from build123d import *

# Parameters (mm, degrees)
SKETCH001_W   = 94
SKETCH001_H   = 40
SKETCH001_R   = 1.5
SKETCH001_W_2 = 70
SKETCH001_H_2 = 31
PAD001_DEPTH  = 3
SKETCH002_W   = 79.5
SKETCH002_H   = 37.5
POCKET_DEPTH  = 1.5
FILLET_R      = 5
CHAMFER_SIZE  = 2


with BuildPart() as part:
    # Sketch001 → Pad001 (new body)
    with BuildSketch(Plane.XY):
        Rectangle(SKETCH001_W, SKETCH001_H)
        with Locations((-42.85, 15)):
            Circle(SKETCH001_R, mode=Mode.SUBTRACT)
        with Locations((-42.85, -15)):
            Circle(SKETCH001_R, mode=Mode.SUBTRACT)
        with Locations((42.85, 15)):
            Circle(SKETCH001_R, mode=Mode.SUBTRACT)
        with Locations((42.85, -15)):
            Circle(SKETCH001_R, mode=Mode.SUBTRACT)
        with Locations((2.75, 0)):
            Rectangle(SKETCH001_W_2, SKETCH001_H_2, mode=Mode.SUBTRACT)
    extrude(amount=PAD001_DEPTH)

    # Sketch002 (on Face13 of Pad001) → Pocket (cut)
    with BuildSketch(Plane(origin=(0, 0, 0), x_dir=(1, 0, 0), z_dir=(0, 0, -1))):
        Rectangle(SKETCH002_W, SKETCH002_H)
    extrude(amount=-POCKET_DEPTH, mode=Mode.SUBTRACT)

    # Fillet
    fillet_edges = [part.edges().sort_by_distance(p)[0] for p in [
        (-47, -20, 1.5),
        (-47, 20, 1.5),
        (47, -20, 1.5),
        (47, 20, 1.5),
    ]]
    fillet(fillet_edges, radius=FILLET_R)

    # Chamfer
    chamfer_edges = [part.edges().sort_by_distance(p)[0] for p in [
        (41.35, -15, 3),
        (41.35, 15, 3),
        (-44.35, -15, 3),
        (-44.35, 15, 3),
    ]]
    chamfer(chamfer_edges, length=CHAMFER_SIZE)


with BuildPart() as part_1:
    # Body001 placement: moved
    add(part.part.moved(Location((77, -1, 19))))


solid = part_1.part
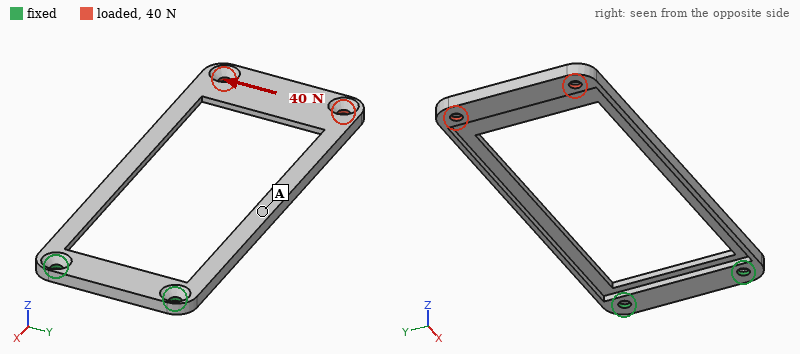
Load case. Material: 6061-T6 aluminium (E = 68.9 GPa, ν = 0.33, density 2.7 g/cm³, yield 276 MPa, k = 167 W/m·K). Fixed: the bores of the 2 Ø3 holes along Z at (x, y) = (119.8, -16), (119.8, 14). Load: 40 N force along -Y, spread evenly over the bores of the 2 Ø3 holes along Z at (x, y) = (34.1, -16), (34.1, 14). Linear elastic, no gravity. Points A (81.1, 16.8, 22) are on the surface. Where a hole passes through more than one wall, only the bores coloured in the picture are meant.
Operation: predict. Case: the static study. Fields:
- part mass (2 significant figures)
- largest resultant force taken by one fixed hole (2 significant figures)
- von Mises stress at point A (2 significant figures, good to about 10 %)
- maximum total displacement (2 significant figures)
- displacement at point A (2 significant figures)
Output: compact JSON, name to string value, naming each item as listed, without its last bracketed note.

{"part mass": "8.9 g", "largest resultant force taken by one fixed hole": "86 N", "von Mises stress at point A": "17 MPa", "maximum total displacement": "1.1 mm", "displacement at point A": "0.45 mm"}
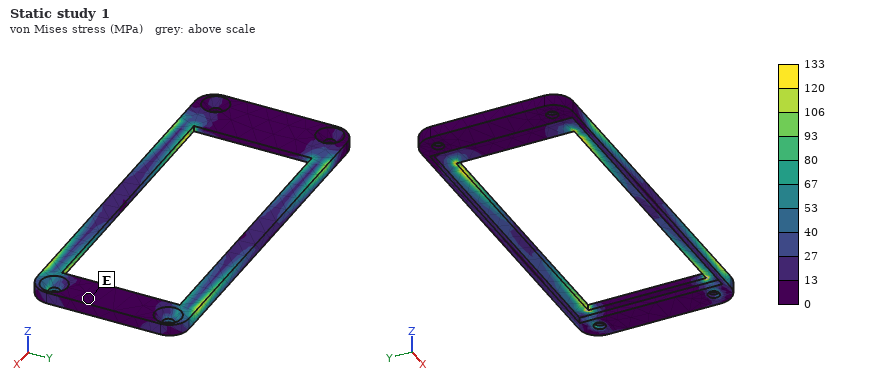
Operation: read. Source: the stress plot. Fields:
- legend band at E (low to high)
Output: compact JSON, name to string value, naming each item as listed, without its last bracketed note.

{"legend band at E": "0 to 13 MPa"}
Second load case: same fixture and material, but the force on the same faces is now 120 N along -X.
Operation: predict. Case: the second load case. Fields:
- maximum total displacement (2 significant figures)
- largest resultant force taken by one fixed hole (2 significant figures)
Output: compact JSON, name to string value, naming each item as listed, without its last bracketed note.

{"maximum total displacement": "1.00 mm", "largest resultant force taken by one fixed hole": "60 N"}
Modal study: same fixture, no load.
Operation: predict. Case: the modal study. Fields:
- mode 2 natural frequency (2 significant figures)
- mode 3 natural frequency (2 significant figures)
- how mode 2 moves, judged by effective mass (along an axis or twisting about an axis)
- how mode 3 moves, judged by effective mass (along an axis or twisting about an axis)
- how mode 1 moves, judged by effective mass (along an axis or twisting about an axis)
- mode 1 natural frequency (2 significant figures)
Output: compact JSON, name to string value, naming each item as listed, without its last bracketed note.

{"mode 2 natural frequency": "440 Hz", "mode 3 natural frequency": "620 Hz", "how mode 2 moves, judged by effective mass": "along Y", "how mode 3 moves, judged by effective mass": "along Y", "how mode 1 moves, judged by effective mass": "along Z", "mode 1 natural frequency": "150 Hz"}
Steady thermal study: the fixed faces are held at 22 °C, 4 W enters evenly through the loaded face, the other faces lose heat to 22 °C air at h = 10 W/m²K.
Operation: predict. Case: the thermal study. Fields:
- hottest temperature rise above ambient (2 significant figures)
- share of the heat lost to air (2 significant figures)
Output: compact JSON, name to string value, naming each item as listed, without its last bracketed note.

{"hottest temperature rise above ambient": "73 K", "share of the heat lost to air": "43 %"}
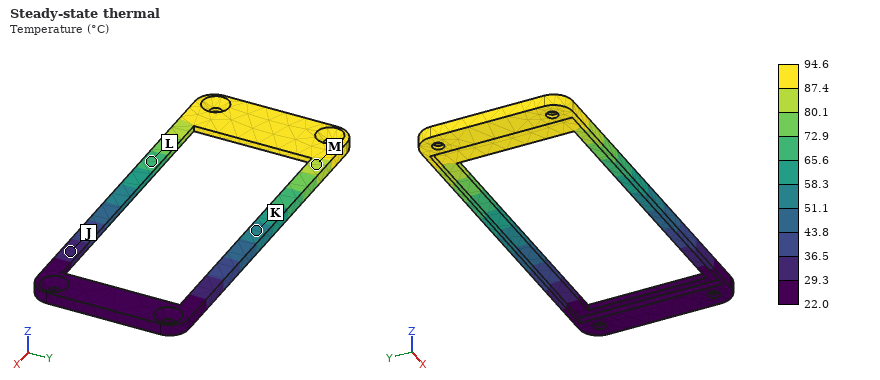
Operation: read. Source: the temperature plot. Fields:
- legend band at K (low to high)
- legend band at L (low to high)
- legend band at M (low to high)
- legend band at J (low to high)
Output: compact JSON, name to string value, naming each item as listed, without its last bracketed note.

{"legend band at K": "51.1 to 58.3 °C", "legend band at L": "65.6 to 72.9 °C", "legend band at M": "80.1 to 87.4 °C", "legend band at J": "29.3 to 36.5 °C"}
